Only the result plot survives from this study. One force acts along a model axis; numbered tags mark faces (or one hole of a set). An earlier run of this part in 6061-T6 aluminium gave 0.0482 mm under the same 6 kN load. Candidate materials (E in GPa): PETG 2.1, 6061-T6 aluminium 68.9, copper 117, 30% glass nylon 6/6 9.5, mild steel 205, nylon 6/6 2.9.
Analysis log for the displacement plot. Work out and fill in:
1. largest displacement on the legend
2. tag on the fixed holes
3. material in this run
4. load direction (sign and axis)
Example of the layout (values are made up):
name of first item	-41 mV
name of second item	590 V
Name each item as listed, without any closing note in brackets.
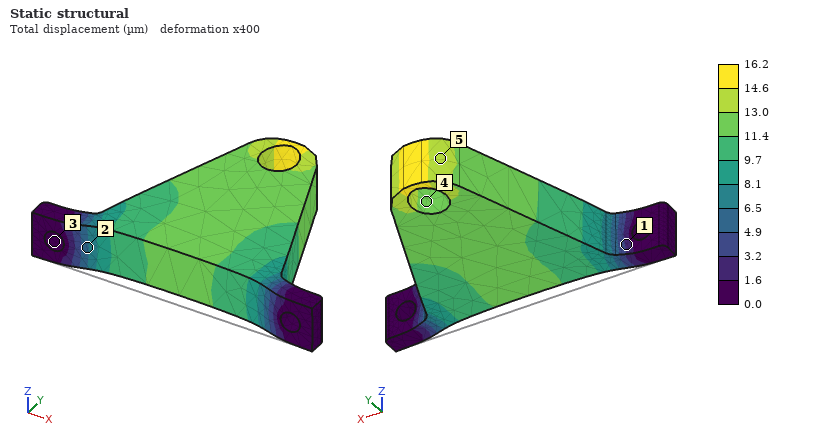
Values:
largest displacement on the legend	16.2 µm
tag on the fixed holes	3
material in this run	mild steel
load direction	+Y
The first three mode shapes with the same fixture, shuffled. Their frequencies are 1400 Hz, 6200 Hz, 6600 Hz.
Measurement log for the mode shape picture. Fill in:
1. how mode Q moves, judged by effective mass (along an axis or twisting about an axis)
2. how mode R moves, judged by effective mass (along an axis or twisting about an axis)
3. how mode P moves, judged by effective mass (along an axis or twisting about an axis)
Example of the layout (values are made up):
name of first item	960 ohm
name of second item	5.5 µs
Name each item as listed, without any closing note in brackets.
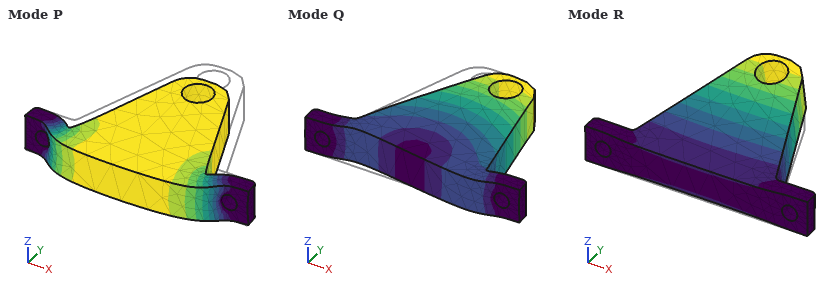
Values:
how mode Q moves, judged by effective mass	along X
how mode R moves, judged by effective mass	along Z
how mode P moves, judged by effective mass	along Y
